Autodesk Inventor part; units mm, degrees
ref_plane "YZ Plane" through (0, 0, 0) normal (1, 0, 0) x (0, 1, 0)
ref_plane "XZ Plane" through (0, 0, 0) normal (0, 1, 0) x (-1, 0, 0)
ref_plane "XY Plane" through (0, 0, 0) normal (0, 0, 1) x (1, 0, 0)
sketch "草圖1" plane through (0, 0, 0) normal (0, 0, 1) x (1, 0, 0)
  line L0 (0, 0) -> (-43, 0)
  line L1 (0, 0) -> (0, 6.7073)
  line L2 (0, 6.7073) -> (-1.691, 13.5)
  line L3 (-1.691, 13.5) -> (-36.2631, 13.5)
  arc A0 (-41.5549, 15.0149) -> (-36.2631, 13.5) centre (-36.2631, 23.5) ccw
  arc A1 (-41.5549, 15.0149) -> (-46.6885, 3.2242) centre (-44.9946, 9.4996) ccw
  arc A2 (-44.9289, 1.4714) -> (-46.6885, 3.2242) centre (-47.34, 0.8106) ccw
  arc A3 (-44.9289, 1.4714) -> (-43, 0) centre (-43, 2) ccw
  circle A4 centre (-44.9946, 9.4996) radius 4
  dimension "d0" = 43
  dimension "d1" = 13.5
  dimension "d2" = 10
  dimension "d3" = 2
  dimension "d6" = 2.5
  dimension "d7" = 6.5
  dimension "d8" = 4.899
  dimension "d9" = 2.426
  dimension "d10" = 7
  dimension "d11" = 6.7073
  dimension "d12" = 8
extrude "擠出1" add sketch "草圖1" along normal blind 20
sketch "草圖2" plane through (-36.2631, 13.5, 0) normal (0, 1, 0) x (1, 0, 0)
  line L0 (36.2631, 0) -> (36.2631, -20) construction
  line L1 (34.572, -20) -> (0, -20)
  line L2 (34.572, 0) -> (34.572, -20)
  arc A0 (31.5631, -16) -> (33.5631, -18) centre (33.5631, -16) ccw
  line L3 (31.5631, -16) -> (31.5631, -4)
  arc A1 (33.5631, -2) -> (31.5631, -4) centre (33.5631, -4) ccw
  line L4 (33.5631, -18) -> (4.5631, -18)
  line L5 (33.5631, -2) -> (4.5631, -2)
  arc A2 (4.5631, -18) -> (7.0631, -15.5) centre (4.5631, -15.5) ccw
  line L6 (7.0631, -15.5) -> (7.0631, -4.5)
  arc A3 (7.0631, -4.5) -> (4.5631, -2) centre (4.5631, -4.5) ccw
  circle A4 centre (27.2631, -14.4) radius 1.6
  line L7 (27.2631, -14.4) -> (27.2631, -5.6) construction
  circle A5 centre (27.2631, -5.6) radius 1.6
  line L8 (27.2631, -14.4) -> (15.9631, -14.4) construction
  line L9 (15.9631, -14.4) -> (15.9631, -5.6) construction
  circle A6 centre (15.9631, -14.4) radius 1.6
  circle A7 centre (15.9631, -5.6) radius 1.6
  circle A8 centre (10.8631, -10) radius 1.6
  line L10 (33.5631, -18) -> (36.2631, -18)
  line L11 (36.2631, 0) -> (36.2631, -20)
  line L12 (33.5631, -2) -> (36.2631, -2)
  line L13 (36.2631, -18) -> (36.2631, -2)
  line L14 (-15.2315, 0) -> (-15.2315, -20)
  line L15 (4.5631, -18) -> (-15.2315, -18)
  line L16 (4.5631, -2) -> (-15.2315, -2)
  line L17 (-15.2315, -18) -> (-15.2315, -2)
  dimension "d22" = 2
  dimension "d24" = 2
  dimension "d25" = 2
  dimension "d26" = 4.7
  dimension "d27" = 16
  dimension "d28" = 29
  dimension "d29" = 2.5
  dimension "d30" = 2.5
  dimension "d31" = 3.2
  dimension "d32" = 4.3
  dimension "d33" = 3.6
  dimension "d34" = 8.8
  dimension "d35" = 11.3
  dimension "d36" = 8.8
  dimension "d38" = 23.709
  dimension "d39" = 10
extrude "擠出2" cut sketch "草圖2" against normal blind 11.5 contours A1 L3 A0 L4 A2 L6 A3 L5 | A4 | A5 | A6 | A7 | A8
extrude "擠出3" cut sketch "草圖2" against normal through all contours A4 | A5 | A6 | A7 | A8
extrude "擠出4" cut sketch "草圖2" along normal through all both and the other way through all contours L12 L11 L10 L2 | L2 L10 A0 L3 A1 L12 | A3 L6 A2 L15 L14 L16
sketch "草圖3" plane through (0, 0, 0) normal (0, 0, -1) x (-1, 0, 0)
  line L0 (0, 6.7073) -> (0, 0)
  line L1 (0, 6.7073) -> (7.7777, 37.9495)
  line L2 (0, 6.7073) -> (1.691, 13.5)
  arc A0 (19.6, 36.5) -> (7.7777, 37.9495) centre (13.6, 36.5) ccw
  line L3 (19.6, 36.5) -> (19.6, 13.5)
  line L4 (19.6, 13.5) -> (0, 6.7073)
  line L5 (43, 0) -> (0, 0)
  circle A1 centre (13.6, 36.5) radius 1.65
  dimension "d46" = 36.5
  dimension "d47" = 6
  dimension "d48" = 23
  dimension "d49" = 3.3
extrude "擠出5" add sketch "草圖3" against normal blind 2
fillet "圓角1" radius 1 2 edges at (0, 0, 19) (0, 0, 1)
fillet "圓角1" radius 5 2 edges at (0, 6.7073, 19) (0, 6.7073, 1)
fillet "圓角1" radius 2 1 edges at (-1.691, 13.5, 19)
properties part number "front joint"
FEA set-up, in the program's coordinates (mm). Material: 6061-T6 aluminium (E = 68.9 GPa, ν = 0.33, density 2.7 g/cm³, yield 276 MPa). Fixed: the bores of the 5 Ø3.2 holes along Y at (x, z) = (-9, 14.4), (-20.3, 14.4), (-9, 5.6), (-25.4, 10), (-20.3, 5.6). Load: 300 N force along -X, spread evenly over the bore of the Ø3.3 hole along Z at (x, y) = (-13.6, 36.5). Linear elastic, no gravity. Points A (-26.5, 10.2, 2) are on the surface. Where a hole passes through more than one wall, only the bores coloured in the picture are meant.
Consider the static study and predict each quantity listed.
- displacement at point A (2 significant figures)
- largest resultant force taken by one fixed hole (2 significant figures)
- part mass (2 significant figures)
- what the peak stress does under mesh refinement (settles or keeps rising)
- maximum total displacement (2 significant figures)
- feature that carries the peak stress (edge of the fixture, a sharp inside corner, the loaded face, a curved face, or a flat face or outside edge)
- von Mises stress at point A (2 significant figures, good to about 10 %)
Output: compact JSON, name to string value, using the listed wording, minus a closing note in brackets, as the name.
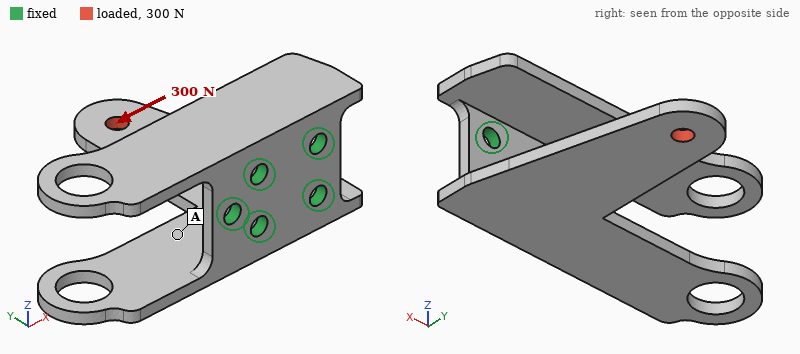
{"displacement at point A": "0.079 mm", "largest resultant force taken by one fixed hole": "780 N", "part mass": "11 g", "what the peak stress does under mesh refinement": "keeps rising", "maximum total displacement": "0.26 mm", "feature that carries the peak stress": "edge of the fixture", "von Mises stress at point A": "41 MPa"}
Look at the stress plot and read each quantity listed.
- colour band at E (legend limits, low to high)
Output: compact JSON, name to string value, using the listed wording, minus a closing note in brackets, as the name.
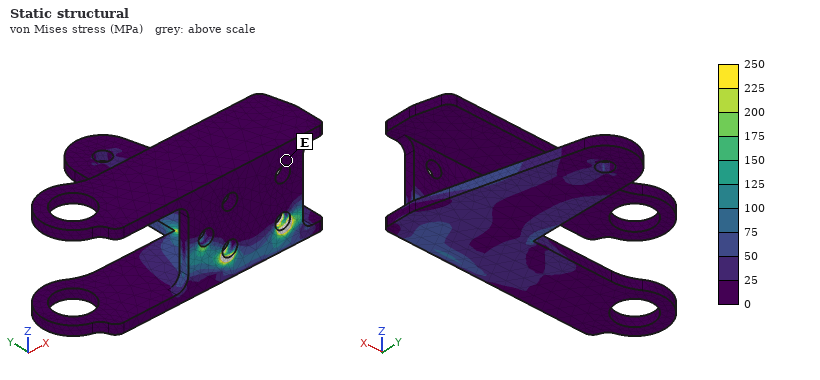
{"colour band at E": "0 to 25 MPa"}
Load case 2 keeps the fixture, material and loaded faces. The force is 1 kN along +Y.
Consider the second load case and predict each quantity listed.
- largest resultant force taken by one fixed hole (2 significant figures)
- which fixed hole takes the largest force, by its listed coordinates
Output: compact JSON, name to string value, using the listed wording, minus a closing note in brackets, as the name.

{"largest resultant force taken by one fixed hole": "600 N", "which fixed hole takes the largest force, by its listed coordinates": "(-9, 5.6)"}
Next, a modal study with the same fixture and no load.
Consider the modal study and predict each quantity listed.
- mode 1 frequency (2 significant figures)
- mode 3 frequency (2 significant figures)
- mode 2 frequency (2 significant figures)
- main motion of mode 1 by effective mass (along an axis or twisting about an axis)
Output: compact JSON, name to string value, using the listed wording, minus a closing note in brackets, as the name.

{"mode 1 frequency": "1200 Hz", "mode 3 frequency": "2800 Hz", "mode 2 frequency": "2800 Hz", "main motion of mode 1 by effective mass": "along Z"}
